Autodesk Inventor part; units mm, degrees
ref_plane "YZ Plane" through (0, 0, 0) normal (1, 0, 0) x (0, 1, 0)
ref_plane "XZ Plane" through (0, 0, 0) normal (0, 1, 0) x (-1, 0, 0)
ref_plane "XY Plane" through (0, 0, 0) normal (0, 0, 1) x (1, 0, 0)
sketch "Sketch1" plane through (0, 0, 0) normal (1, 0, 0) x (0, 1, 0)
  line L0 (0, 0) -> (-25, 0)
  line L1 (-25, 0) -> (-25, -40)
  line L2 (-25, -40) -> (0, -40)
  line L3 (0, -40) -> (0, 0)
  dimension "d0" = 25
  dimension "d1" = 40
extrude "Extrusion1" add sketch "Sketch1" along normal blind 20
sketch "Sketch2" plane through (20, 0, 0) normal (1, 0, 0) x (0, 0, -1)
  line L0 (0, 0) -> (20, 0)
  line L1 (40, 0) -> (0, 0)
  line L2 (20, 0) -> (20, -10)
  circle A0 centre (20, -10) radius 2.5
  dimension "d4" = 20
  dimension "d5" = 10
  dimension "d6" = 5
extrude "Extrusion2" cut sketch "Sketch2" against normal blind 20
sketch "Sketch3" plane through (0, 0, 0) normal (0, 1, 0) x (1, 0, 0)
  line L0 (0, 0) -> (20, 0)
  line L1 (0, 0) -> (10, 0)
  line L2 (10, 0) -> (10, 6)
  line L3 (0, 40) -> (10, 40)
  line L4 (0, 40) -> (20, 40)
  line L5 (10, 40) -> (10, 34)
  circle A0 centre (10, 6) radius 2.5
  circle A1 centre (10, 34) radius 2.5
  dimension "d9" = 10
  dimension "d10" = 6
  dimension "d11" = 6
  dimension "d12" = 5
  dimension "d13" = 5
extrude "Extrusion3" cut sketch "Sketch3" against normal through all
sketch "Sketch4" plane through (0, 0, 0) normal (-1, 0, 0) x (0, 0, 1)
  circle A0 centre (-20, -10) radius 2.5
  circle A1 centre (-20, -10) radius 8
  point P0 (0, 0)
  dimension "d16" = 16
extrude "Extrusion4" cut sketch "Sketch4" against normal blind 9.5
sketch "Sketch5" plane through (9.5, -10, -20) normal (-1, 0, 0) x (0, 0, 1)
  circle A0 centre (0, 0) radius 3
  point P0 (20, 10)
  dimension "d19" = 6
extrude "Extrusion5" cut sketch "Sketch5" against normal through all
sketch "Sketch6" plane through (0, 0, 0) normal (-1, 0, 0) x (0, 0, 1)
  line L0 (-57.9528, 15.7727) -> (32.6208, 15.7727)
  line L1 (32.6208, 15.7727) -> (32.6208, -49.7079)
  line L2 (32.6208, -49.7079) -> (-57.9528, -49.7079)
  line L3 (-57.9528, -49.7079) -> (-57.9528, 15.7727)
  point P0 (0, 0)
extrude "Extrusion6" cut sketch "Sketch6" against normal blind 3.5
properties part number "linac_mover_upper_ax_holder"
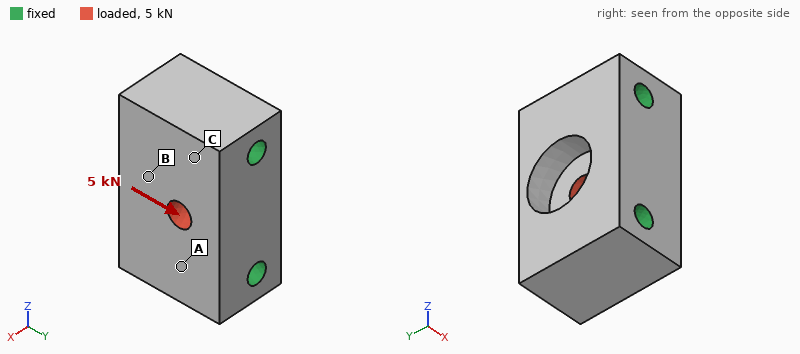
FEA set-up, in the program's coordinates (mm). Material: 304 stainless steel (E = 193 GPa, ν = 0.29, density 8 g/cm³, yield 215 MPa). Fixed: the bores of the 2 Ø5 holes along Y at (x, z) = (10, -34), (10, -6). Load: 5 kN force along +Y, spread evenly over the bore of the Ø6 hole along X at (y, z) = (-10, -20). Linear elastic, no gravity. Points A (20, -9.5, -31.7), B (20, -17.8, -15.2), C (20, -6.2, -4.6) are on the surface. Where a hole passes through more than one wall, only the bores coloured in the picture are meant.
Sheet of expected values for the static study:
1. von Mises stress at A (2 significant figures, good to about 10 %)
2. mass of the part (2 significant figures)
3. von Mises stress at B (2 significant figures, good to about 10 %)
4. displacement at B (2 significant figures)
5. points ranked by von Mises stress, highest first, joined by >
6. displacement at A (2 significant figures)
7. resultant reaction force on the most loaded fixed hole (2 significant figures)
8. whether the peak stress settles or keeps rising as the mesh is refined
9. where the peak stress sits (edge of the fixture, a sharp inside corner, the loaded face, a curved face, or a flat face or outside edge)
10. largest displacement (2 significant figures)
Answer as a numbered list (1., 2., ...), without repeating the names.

1. 8.5 MPa
2. 110 g
3. 16 MPa
4. 1.4 µm
5. B > A > C
6. 0.58 µm
7. 2.5 kN
8. keeps rising
9. edge of the fixture
10. 2.6 µm
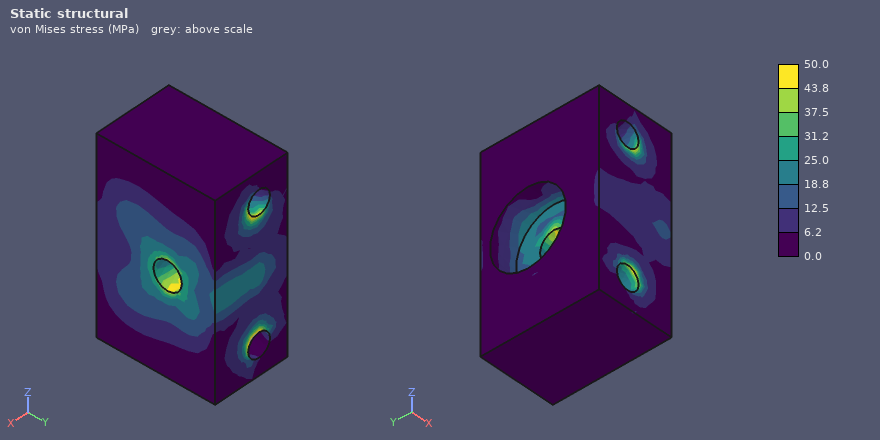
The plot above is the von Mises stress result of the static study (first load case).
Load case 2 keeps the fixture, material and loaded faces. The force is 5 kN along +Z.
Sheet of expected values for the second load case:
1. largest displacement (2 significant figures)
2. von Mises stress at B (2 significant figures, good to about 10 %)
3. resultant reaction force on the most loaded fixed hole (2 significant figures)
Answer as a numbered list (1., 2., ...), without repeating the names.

1. 1.3 µm
2. 5.8 MPa
3. 2.6 kN
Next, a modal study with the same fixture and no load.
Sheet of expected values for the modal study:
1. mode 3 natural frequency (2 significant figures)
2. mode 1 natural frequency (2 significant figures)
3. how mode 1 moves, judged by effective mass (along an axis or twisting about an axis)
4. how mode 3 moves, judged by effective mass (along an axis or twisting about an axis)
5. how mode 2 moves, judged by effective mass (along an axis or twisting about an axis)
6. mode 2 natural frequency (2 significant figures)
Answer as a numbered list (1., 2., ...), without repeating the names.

1. 53 kHz
2. 44 kHz
3. along X
4. along Y
5. along Y
6. 48 kHz
